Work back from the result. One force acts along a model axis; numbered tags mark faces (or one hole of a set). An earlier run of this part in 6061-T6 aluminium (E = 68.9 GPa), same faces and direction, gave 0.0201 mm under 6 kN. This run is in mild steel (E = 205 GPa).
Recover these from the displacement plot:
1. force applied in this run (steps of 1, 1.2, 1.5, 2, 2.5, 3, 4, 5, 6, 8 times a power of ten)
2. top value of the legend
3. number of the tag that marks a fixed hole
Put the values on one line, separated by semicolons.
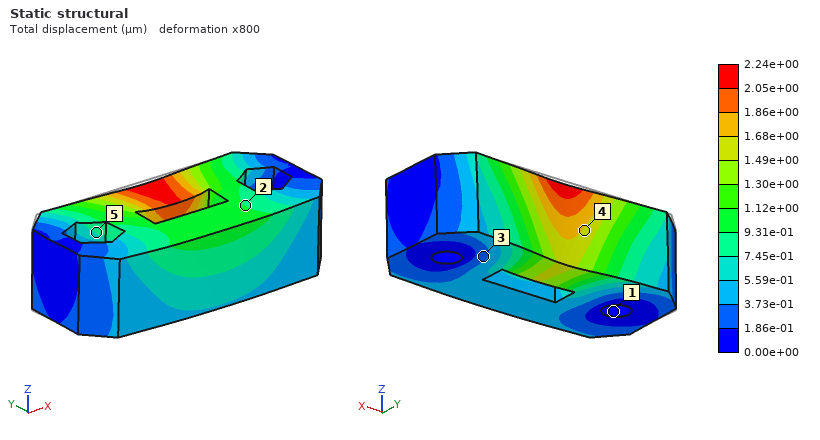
2 kN; 2.24e+00 µm; 1
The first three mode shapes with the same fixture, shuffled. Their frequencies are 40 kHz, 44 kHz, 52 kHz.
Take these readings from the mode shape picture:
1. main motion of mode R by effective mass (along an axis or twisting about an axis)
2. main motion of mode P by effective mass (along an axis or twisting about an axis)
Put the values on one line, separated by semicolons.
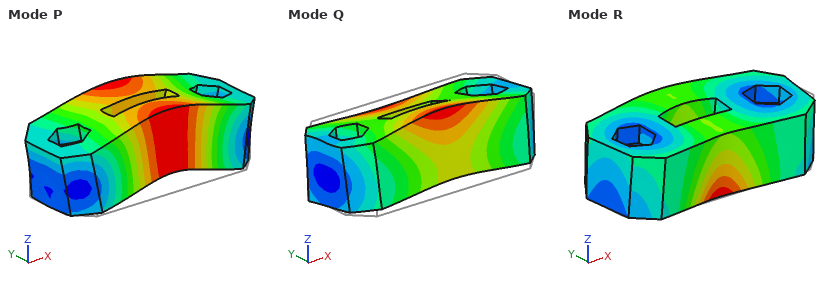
along Y; along Z
